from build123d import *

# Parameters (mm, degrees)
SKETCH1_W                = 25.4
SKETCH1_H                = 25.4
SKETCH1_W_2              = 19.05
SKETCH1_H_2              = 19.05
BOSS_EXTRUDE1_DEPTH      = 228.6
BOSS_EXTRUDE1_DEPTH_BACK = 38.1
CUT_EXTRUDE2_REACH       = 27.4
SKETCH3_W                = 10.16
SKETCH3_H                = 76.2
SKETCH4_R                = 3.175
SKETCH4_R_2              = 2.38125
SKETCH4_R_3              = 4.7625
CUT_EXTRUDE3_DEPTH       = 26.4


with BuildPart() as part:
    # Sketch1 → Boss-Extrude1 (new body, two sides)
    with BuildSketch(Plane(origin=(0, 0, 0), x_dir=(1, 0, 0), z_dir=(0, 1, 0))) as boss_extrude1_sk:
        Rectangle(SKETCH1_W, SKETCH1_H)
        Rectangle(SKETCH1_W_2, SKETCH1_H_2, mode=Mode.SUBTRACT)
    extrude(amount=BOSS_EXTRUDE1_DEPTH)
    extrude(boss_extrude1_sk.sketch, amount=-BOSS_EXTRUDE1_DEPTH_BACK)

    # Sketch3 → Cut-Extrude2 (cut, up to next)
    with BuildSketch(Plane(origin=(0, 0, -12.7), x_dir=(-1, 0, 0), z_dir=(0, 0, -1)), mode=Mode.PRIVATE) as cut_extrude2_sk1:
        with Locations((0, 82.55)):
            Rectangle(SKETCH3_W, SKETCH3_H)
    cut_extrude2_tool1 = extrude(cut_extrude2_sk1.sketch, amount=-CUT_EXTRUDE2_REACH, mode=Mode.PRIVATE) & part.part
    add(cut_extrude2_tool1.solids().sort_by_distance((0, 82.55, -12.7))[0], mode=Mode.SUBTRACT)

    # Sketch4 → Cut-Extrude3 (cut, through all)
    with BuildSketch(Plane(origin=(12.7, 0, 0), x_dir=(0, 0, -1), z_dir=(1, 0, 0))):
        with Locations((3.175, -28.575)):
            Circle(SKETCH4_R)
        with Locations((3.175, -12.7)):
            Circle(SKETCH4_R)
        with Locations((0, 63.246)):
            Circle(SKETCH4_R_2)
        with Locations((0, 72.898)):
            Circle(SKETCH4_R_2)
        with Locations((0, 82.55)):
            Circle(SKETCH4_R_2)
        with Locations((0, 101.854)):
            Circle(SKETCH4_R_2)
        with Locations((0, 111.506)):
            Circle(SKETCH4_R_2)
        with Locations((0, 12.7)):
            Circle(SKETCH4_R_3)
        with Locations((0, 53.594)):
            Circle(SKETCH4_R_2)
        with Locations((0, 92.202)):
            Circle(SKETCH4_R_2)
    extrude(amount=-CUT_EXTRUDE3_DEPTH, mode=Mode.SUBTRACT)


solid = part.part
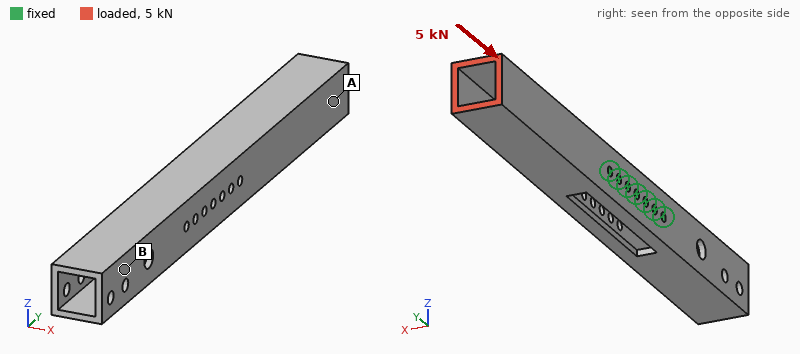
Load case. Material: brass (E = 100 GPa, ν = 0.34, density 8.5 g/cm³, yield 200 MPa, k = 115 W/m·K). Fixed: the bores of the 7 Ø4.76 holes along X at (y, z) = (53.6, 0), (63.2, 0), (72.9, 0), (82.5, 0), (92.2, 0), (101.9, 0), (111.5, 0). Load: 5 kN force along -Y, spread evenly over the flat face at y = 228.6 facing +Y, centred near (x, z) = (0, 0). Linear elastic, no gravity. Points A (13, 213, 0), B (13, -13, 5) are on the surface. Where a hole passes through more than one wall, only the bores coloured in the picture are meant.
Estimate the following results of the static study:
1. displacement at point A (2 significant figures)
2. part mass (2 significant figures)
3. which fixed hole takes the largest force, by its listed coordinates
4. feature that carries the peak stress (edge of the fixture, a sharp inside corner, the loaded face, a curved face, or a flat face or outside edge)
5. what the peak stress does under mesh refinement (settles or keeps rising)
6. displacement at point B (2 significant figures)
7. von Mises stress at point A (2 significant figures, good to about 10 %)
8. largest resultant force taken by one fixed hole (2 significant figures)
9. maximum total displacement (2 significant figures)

0.21 mm
600 g
(111.5, 0)
edge of the fixture
keeps rising
0.13 mm
18 MPa
1.9 kN
0.25 mm
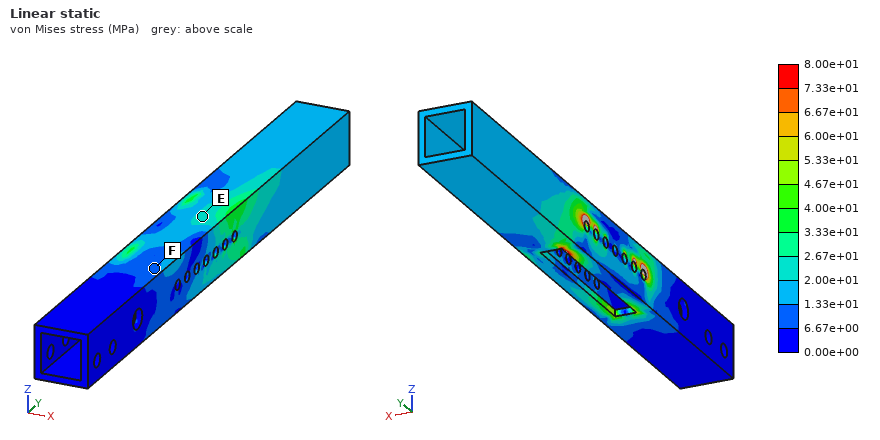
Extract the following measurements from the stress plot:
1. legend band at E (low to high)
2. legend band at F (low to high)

2.00e+01 to 2.67e+01 MPa
6.67e+00 to 1.33e+01 MPa
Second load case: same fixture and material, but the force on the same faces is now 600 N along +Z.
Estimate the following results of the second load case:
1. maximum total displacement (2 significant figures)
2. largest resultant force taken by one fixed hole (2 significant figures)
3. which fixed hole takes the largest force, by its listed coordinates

0.37 mm
2.4 kN
(111.5, 0)
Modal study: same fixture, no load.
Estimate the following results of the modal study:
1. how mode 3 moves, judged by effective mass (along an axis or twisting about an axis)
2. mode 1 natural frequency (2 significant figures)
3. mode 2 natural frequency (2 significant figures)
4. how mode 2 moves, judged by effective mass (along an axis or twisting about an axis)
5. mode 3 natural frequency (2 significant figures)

along Z
520 Hz
720 Hz
along Z
910 Hz
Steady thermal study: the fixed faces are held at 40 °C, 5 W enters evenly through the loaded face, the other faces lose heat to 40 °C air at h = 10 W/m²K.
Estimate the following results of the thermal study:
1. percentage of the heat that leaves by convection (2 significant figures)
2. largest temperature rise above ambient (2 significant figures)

37 %
16 K
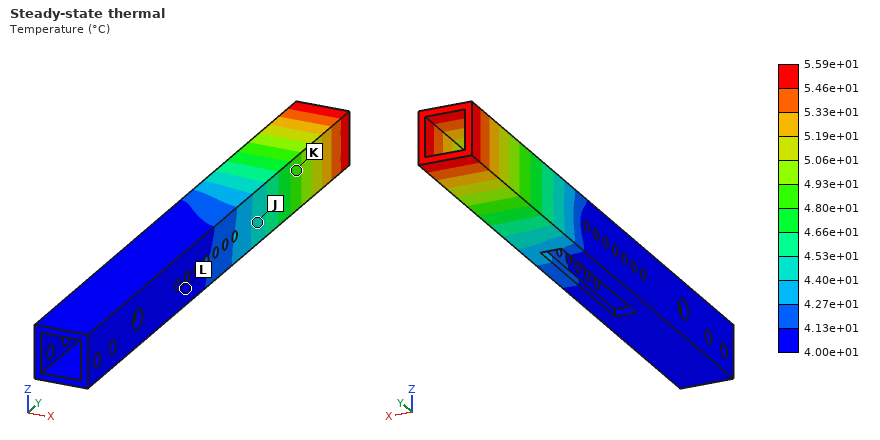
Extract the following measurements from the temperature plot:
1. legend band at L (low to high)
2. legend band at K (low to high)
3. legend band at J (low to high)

4.00e+01 to 4.13e+01 °C
4.80e+01 to 4.93e+01 °C
4.40e+01 to 4.53e+01 °C
